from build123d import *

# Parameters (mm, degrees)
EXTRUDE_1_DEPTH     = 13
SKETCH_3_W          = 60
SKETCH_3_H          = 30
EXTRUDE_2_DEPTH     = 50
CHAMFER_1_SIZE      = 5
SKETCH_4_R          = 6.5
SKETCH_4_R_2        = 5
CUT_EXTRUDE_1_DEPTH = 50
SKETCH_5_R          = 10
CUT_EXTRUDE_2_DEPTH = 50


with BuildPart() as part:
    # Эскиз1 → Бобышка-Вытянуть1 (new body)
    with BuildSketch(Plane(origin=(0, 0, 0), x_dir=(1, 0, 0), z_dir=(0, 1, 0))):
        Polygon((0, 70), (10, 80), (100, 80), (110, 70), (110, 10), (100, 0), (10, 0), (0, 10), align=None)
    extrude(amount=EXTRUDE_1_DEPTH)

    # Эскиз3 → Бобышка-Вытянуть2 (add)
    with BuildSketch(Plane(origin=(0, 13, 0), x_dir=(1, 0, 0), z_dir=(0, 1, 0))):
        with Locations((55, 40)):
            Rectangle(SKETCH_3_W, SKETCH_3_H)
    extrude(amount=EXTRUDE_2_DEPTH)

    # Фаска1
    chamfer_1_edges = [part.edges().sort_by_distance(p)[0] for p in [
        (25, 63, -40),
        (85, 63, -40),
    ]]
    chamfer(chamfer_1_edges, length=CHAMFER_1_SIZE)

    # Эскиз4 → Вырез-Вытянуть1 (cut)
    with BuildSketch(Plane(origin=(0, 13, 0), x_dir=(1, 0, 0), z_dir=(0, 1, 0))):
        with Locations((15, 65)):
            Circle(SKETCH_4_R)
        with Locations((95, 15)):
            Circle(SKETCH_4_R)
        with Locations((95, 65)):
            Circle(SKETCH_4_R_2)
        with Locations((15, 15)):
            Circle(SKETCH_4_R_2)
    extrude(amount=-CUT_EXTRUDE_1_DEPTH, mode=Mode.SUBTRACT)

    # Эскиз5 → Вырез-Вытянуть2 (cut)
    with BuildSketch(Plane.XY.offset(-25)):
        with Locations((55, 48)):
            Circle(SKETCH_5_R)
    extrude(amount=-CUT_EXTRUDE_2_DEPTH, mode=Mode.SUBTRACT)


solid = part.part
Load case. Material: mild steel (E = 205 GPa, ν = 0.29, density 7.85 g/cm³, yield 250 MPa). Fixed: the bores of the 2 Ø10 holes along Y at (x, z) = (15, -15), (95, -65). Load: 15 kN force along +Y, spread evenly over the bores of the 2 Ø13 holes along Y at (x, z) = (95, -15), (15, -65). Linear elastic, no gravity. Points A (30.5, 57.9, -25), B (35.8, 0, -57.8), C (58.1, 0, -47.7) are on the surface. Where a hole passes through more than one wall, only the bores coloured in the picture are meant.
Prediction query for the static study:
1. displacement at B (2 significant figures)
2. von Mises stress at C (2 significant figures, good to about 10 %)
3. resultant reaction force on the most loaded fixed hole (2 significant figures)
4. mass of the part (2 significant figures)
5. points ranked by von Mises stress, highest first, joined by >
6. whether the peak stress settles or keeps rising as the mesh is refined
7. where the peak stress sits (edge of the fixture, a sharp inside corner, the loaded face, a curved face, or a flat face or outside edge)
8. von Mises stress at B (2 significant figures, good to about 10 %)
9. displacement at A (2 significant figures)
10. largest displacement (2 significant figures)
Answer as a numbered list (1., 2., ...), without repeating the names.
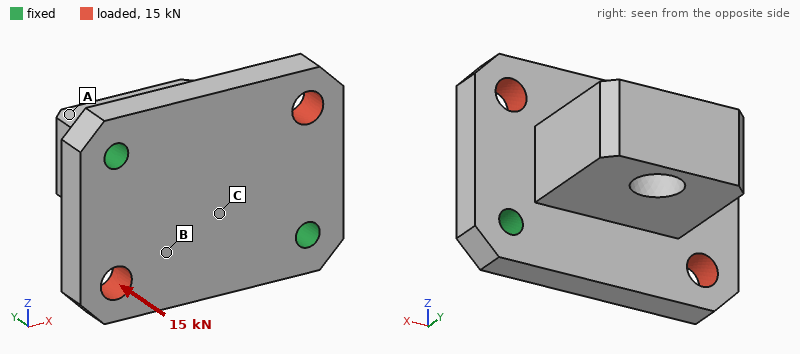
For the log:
1. 23 µm
2. 42 MPa
3. 8.0 kN
4. 1.5 kg
5. B > C > A
6. keeps rising
7. edge of the fixture
8. 73 MPa
9. 16 µm
10. 75 µm
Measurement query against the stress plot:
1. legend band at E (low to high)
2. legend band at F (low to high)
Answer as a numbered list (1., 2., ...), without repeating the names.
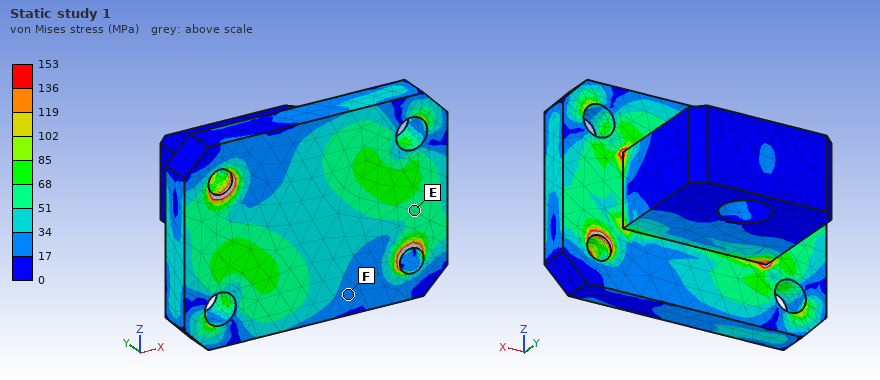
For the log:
1. 51 to 68 MPa
2. 17 to 34 MPa
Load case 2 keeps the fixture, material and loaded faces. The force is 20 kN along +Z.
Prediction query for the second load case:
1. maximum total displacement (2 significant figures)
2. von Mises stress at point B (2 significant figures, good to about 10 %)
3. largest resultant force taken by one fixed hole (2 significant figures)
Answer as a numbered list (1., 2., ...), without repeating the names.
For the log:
1. 8.8 µm
2. 7.5 MPa
3. 10 kN
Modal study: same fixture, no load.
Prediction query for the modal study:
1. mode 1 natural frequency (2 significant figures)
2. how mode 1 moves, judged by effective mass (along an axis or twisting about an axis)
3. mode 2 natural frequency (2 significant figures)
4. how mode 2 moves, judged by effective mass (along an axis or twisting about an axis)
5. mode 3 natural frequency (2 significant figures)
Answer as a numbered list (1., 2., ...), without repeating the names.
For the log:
1. 2000 Hz
2. along Z
3. 4500 Hz
4. along Y
5. 5600 Hz
